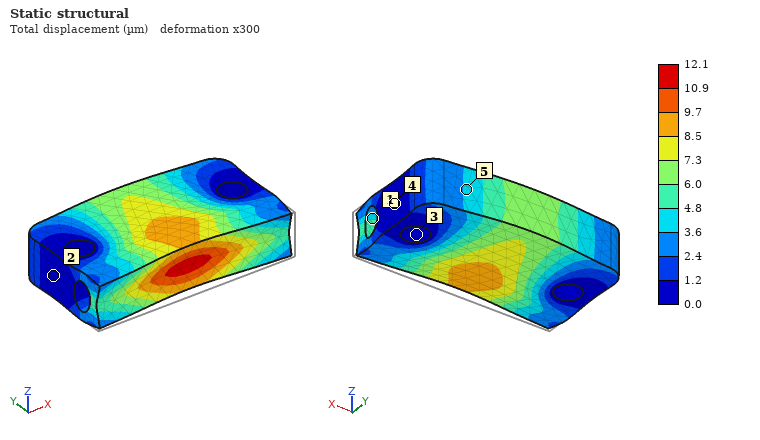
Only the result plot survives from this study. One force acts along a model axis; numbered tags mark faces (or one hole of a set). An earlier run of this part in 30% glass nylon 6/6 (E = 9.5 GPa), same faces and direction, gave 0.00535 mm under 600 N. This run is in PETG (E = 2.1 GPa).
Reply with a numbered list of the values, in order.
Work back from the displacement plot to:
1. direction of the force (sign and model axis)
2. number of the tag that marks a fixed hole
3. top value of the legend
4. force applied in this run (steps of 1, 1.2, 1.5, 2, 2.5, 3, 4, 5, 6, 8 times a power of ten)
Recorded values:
1. +Y
2. 3
3. 12.1 µm
4. 300 N
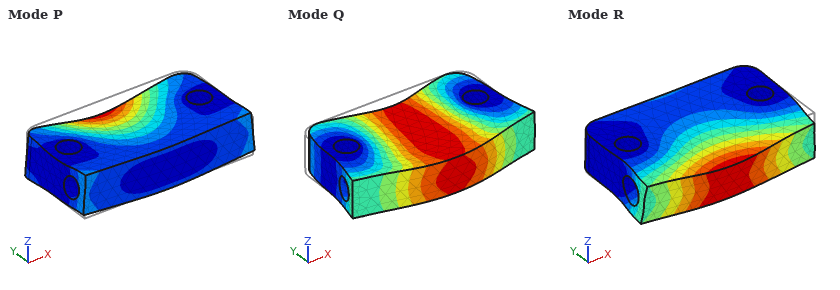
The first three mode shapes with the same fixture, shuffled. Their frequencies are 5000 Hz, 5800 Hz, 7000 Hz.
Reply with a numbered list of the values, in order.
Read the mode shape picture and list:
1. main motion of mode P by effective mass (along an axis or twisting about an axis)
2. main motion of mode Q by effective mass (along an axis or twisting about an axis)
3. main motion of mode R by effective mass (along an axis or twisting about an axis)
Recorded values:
1. along Z
2. along Y
3. along Z
